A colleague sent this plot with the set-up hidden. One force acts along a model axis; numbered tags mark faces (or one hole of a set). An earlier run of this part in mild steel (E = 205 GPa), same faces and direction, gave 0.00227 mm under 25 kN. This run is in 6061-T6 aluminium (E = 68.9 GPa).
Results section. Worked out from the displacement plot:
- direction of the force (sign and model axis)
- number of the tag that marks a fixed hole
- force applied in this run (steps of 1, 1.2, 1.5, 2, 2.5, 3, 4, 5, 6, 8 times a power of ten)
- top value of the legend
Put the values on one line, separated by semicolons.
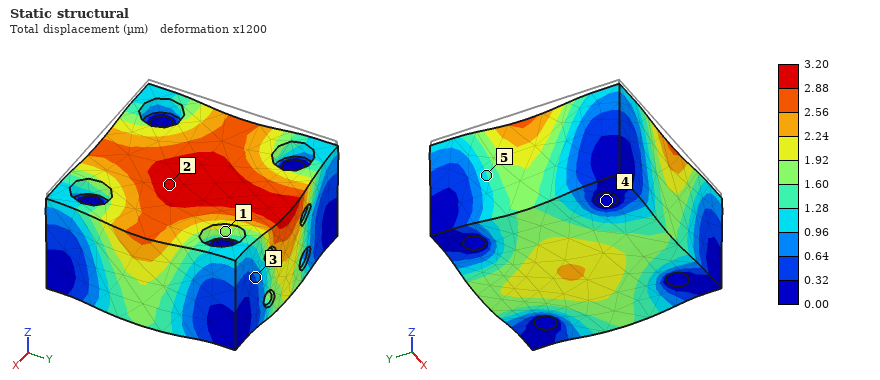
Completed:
-Z; 4; 12 kN; 3.20 µm
